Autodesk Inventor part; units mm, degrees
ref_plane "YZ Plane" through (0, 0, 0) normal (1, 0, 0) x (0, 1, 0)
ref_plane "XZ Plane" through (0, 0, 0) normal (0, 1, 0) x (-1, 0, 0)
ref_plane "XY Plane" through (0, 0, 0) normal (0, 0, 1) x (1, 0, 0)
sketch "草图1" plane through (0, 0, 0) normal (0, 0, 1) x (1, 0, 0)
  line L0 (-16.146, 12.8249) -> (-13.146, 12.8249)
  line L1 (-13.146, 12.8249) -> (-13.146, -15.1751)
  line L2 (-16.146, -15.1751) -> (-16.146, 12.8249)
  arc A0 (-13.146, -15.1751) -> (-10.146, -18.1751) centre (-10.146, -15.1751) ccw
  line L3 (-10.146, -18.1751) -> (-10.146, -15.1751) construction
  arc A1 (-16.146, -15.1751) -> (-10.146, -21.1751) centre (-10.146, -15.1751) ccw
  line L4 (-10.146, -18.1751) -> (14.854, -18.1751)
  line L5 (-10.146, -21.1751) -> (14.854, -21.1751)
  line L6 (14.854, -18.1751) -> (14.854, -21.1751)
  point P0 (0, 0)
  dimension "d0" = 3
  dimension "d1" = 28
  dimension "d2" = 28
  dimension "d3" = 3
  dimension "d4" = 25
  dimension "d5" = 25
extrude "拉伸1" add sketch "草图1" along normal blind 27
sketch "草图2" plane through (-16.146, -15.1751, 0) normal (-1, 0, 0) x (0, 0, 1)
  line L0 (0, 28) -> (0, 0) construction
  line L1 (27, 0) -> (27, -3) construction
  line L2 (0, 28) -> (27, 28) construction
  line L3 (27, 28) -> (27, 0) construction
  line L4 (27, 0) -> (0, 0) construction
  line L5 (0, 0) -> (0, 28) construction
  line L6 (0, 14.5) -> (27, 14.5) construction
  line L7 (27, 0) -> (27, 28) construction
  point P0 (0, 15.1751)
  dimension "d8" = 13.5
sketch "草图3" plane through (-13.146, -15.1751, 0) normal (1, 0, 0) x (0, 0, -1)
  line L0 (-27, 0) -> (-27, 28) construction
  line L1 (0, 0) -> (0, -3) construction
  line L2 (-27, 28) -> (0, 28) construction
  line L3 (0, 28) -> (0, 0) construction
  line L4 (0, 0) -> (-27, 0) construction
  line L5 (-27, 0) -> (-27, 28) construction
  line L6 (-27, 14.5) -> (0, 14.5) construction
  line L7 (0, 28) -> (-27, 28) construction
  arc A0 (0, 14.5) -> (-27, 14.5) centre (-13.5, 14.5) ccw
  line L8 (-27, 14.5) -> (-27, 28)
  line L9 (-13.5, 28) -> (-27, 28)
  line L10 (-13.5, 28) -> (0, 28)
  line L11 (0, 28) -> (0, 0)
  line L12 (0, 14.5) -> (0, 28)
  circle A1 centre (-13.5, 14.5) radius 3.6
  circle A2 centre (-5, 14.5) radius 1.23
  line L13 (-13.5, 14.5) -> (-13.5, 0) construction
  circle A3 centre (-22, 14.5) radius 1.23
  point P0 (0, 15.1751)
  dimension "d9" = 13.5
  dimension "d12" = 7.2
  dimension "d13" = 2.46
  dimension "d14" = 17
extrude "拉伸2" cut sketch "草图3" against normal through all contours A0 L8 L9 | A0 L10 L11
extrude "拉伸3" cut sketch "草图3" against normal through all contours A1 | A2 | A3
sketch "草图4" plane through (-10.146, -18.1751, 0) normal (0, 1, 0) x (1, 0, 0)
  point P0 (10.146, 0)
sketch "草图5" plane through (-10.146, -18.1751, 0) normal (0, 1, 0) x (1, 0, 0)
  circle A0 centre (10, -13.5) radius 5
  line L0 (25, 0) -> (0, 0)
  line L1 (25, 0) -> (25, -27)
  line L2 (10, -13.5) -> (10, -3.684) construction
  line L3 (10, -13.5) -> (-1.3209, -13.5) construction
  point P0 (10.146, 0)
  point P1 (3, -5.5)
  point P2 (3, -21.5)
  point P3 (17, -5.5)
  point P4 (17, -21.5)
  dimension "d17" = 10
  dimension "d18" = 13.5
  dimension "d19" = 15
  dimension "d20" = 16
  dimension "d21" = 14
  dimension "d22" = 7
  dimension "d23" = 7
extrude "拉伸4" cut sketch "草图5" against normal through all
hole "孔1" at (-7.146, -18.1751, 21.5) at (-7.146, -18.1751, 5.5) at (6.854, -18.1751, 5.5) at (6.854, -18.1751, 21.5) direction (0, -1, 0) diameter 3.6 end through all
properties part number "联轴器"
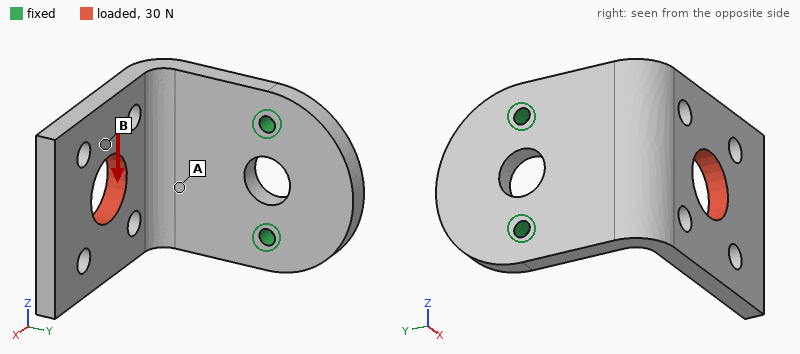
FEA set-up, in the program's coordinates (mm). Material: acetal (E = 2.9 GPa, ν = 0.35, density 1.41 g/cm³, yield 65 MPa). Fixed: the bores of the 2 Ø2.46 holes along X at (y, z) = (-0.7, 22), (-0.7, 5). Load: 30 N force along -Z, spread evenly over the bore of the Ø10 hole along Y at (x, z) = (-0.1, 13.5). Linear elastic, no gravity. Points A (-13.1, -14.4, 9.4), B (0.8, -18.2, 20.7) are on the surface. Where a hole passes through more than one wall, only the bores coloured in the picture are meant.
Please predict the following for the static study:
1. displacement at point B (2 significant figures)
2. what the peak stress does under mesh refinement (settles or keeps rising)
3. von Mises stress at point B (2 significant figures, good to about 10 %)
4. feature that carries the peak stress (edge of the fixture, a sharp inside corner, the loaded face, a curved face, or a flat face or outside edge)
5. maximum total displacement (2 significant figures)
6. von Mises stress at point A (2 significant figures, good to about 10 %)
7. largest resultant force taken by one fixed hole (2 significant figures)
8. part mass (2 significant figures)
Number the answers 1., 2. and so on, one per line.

1. 0.33 mm
2. keeps rising
3. 1.6 MPa
4. edge of the fixture
5. 0.61 mm
6. 7.3 MPa
7. 40 N
8. 5.8 g
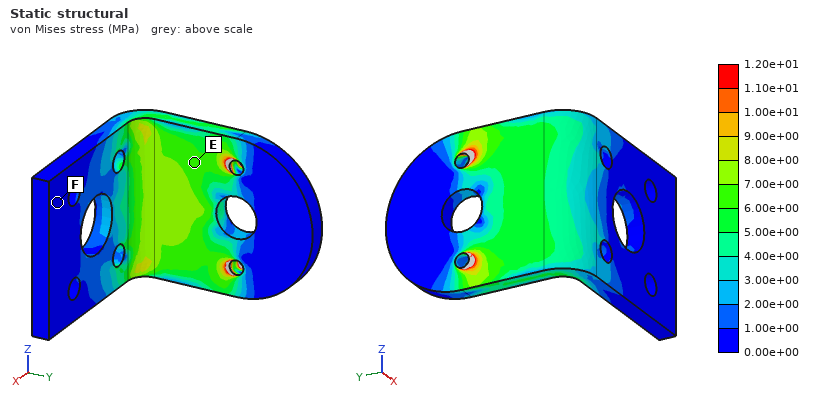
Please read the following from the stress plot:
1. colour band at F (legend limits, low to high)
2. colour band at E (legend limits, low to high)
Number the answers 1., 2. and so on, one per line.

1. 0.00e+00 to 1.00e+00 MPa
2. 6.00e+00 to 7.00e+00 MPa
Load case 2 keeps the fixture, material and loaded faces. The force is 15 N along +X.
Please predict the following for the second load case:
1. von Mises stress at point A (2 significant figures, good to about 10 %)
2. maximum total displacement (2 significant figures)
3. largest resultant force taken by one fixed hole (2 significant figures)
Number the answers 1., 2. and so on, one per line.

1. 1.9 MPa
2. 0.56 mm
3. 7.5 N
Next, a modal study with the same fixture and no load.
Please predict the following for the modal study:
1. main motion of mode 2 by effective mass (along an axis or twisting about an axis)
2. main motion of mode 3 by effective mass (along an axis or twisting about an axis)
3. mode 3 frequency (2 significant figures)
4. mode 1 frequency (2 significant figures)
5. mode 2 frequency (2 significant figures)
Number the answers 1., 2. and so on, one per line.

1. along Z
2. along X
3. 1200 Hz
4. 400 Hz
5. 730 Hz
